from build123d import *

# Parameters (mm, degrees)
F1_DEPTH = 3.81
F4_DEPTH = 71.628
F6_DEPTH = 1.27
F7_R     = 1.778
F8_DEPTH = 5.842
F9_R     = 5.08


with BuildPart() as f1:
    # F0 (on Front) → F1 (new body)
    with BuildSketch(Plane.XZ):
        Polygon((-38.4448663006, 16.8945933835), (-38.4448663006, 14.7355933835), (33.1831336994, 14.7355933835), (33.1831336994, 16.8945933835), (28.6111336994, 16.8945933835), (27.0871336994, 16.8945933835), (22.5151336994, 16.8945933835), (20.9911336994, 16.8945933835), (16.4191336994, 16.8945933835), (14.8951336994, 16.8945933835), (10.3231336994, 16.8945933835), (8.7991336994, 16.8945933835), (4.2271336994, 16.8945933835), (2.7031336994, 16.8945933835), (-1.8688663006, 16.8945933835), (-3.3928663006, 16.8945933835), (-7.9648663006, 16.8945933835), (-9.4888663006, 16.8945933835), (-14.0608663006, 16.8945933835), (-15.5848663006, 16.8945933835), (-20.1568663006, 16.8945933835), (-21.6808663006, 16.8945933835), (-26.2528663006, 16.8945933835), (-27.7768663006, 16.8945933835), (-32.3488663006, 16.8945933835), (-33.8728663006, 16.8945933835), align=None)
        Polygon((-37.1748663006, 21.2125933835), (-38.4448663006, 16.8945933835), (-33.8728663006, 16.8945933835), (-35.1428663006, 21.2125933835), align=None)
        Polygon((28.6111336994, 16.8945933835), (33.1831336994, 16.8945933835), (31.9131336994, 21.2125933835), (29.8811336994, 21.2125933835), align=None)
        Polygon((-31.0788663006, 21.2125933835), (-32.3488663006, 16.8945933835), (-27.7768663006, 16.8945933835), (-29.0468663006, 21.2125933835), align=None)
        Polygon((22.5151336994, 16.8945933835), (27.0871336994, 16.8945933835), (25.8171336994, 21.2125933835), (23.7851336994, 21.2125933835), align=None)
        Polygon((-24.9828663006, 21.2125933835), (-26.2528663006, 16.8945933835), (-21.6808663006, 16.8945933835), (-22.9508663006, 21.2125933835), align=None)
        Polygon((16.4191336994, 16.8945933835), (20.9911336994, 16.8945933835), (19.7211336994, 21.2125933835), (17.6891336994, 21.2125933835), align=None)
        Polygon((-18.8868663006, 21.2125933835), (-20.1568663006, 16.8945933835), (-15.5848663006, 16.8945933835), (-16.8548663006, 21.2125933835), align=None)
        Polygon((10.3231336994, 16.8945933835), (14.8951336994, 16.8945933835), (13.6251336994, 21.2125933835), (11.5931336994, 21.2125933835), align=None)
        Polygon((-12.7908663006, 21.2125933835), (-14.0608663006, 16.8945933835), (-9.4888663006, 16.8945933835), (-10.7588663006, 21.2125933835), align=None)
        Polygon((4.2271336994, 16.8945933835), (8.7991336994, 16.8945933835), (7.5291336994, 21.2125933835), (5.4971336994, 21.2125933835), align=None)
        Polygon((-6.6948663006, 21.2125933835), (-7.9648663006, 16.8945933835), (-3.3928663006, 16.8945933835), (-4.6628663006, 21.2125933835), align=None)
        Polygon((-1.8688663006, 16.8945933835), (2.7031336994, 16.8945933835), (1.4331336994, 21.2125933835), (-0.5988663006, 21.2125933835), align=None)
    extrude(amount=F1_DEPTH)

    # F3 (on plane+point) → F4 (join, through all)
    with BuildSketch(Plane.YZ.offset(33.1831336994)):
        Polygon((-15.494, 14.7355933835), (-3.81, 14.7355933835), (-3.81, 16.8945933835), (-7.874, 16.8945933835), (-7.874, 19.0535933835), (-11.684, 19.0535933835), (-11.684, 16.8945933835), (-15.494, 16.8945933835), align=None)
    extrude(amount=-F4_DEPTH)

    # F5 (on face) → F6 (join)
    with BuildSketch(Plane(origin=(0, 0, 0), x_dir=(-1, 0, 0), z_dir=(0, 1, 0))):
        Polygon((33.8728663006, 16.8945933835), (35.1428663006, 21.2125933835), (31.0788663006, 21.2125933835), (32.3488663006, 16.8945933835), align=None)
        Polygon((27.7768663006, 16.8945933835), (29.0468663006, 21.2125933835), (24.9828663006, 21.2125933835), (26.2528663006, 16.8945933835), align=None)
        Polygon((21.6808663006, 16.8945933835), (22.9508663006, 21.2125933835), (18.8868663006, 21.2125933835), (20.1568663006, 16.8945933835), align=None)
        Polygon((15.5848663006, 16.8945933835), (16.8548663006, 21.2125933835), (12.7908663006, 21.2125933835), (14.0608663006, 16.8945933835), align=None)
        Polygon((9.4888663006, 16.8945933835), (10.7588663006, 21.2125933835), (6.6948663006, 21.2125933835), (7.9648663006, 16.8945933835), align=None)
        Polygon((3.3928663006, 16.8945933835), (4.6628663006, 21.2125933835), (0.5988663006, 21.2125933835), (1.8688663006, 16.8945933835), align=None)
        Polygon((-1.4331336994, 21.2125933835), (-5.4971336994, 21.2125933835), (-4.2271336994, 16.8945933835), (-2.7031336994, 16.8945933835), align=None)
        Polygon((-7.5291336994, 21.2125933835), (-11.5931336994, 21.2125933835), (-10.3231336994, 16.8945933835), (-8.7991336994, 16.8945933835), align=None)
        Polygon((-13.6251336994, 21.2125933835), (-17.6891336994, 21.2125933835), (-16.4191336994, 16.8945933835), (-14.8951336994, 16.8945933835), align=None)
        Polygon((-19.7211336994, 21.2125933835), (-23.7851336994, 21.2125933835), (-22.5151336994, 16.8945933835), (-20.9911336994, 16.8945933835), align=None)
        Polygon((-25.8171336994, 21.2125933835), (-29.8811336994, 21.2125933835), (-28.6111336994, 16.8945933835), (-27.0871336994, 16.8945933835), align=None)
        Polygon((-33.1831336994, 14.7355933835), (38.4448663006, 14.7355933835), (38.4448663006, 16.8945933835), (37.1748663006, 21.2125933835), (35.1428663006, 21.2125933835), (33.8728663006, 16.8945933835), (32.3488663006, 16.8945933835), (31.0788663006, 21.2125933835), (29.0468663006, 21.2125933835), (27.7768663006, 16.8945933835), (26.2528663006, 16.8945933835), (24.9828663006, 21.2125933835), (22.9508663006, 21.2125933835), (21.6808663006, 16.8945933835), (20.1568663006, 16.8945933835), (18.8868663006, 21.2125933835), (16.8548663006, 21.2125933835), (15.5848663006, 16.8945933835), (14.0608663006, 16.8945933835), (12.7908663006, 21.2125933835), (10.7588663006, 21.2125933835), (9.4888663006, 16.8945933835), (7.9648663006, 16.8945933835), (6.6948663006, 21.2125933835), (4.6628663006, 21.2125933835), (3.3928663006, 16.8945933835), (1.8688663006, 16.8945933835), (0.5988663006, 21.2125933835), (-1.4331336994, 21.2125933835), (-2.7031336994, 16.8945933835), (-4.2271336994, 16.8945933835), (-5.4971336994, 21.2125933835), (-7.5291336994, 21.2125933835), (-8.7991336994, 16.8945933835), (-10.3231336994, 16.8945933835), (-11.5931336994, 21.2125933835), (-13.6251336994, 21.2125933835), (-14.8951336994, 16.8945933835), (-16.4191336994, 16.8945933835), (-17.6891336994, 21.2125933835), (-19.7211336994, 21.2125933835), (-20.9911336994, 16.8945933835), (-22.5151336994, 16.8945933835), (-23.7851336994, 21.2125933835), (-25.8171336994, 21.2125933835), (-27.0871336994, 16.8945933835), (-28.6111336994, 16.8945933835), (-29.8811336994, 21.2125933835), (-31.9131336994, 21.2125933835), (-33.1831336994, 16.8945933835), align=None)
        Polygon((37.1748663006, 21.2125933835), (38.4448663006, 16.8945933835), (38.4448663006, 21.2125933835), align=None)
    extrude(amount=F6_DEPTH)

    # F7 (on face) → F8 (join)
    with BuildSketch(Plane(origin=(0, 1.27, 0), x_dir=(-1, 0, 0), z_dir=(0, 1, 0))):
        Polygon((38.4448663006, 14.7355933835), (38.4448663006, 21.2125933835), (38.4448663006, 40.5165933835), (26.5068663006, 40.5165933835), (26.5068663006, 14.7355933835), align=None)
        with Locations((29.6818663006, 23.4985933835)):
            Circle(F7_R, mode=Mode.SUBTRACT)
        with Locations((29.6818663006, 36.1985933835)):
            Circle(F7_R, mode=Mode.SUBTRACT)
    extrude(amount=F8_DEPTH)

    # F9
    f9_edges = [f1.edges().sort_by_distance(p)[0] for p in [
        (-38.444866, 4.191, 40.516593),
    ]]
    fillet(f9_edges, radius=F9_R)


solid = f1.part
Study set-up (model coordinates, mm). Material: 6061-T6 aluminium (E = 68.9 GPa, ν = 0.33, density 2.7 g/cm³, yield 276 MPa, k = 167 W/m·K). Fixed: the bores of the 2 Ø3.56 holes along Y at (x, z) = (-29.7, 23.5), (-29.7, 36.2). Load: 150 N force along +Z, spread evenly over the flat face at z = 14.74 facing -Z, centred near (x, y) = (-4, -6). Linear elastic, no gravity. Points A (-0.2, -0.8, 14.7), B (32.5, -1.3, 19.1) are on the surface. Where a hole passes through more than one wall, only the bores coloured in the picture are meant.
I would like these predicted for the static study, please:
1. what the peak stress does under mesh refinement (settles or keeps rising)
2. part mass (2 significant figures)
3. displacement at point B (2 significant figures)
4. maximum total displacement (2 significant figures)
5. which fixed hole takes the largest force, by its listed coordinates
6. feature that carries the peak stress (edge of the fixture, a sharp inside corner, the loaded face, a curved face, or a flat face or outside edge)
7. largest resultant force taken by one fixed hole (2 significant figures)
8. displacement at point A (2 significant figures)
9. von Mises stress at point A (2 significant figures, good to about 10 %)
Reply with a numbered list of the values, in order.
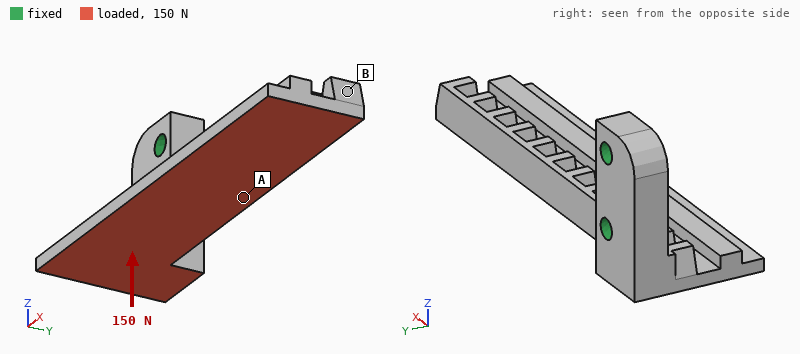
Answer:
1. keeps rising
2. 16 g
3. 0.70 mm
4. 0.79 mm
5. (-29.7, 23.5)
6. a sharp inside corner
7. 380 N
8. 0.24 mm
9. 26 MPa
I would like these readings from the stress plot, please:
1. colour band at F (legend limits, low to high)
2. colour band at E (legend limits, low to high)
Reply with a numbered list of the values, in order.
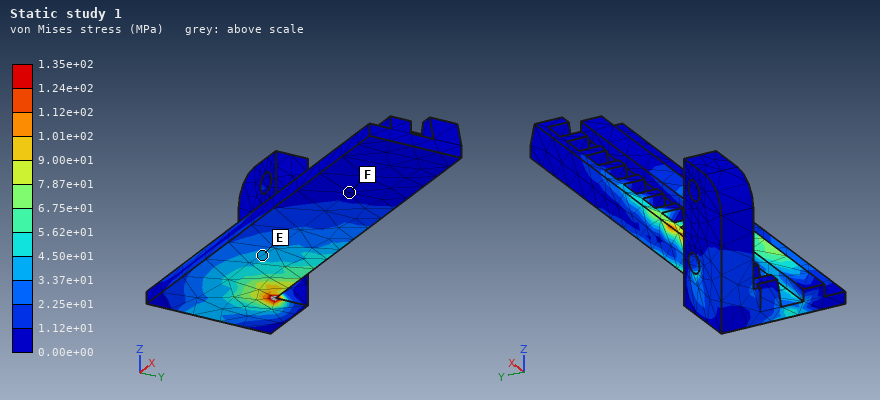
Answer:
1. 0.00e+00 to 1.12e+01 MPa
2. 3.37e+01 to 4.50e+01 MPa
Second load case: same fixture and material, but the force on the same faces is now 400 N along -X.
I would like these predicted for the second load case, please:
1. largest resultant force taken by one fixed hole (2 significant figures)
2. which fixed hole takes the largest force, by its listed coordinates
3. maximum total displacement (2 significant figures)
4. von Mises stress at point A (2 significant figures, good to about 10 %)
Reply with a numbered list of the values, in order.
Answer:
1. 560 N
2. (-29.7, 23.5)
3. 0.20 mm
4. 10 MPa
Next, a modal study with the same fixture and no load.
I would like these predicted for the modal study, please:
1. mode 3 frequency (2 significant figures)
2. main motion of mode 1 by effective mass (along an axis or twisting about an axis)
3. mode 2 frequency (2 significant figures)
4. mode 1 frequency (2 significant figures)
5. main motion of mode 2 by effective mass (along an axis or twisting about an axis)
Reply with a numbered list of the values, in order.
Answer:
1. 3300 Hz
2. along Z
3. 1500 Hz
4. 810 Hz
5. along Y
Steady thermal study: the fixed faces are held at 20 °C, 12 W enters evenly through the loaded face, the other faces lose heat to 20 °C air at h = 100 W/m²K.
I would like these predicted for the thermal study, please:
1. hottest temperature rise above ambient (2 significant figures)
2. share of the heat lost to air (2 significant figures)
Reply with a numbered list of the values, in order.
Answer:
1. 24 K
2. 40 %
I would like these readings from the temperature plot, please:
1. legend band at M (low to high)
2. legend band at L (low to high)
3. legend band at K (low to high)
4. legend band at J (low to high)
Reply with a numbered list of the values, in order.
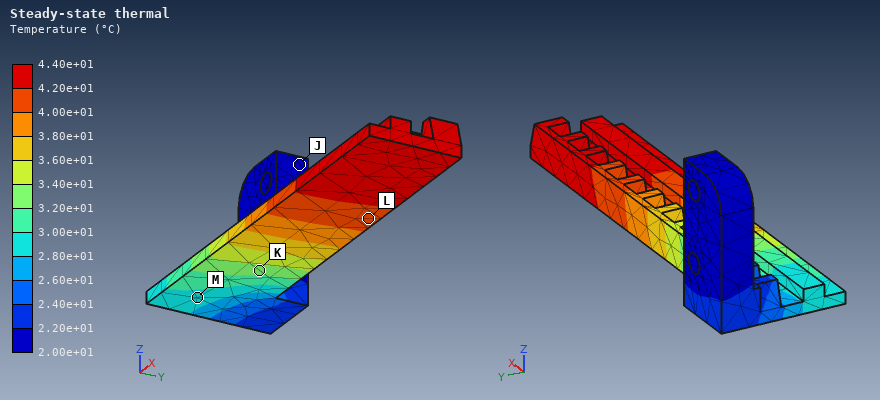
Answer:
1. 2.80e+01 to 3.00e+01 °C
2. 4.00e+01 to 4.20e+01 °C
3. 3.20e+01 to 3.40e+01 °C
4. 2.00e+01 to 2.20e+01 °C
